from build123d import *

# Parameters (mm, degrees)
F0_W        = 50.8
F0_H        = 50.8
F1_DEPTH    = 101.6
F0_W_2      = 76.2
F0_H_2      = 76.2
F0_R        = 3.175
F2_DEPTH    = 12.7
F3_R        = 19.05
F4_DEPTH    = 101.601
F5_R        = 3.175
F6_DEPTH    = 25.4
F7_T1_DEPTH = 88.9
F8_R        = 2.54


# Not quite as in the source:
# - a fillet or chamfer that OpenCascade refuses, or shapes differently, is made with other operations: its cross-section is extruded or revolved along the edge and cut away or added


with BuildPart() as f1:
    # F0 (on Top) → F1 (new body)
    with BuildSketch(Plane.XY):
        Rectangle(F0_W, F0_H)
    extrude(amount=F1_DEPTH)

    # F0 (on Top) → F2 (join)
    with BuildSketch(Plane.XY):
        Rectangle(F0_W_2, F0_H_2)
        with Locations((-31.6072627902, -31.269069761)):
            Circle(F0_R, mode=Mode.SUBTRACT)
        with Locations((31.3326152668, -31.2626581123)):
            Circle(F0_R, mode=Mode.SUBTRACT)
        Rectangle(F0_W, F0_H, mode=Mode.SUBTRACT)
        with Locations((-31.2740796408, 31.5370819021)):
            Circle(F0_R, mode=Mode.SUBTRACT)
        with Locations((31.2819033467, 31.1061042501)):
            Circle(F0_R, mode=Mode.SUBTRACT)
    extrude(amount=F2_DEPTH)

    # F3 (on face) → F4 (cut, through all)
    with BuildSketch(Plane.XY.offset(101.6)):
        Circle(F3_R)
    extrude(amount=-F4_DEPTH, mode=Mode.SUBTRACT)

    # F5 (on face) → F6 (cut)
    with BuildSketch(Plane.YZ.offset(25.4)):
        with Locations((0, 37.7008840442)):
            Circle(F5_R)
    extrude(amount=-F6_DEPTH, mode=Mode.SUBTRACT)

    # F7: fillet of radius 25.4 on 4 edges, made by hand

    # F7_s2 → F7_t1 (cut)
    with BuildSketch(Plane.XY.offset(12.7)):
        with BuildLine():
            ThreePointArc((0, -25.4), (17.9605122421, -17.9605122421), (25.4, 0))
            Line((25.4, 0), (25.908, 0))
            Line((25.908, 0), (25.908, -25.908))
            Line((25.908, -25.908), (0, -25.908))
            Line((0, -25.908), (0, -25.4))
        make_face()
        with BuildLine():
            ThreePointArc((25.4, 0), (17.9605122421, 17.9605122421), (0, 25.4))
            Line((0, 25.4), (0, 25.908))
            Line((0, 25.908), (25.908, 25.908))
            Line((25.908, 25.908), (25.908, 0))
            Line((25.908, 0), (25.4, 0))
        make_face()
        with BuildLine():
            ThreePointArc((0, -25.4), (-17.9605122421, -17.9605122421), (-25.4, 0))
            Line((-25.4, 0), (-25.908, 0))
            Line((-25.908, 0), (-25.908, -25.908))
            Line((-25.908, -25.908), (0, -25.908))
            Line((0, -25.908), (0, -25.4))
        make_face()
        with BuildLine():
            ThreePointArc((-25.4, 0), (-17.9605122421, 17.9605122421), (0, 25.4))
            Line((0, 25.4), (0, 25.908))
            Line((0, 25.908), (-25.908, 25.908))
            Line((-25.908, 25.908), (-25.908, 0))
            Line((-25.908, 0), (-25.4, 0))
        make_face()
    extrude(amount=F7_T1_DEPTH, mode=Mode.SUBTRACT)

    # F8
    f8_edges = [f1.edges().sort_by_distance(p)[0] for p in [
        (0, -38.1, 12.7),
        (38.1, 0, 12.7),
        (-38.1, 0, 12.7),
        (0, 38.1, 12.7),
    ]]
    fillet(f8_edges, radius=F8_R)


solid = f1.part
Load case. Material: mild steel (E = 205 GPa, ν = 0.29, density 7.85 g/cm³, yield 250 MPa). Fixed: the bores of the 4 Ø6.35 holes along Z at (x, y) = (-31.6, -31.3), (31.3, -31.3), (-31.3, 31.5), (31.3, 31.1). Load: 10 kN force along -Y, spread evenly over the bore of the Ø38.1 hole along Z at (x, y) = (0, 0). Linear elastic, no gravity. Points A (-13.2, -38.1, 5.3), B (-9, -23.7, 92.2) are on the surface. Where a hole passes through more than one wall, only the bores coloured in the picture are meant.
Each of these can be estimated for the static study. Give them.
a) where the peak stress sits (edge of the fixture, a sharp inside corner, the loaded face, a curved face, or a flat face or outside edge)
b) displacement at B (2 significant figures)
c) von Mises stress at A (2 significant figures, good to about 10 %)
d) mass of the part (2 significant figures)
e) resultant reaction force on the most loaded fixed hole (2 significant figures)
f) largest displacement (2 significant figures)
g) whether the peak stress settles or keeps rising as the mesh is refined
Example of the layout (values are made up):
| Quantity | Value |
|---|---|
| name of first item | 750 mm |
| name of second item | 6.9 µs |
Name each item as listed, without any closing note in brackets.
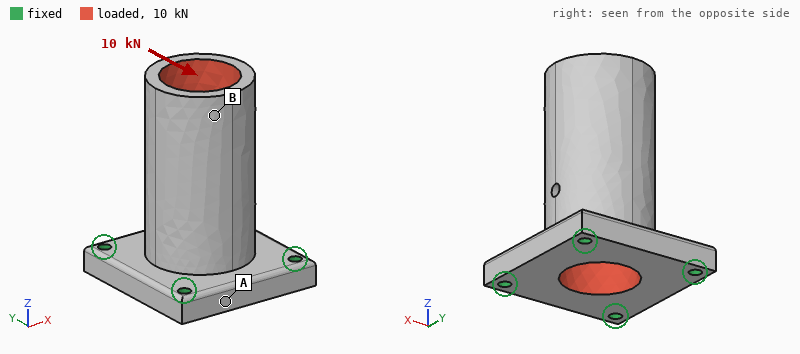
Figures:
| Quantity | Value |
|---|---|
| where the peak stress sits | edge of the fixture |
| displacement at B | 67 µm |
| von Mises stress at A | 26 MPa |
| mass of the part | 1.1 kg |
| resultant reaction force on the most loaded fixed hole | 4.9 kN |
| largest displacement | 75 µm |
| whether the peak stress settles or keeps rising as the mesh is refined | keeps rising |
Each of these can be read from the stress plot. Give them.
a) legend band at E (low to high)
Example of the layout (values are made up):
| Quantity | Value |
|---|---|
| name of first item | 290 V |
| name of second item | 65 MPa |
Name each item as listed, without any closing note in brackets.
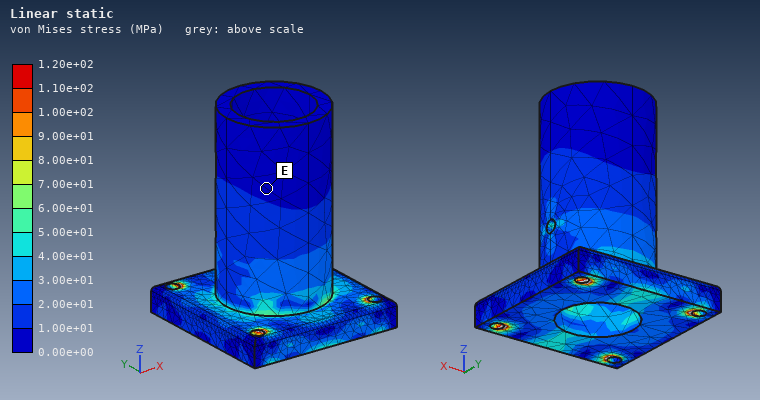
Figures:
| Quantity | Value |
|---|---|
| legend band at E | 0.00e+00 to 1.00e+01 MPa |
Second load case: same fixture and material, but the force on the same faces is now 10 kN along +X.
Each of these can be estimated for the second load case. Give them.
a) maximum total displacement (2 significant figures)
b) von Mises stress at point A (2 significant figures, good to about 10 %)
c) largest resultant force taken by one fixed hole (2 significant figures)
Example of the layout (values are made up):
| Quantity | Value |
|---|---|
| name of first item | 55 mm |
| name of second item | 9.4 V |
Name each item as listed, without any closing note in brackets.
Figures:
| Quantity | Value |
|---|---|
| maximum total displacement | 75 µm |
| von Mises stress at point A | 11 MPa |
| largest resultant force taken by one fixed hole | 5.0 kN |
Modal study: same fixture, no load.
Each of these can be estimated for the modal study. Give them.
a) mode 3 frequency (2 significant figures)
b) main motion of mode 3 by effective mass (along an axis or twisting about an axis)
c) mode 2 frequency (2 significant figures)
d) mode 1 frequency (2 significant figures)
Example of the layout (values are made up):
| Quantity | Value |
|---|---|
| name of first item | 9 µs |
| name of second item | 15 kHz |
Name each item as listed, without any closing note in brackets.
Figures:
| Quantity | Value |
|---|---|
| mode 3 frequency | 6300 Hz |
| main motion of mode 3 by effective mass | along Z |
| mode 2 frequency | 2600 Hz |
| mode 1 frequency | 2600 Hz |
